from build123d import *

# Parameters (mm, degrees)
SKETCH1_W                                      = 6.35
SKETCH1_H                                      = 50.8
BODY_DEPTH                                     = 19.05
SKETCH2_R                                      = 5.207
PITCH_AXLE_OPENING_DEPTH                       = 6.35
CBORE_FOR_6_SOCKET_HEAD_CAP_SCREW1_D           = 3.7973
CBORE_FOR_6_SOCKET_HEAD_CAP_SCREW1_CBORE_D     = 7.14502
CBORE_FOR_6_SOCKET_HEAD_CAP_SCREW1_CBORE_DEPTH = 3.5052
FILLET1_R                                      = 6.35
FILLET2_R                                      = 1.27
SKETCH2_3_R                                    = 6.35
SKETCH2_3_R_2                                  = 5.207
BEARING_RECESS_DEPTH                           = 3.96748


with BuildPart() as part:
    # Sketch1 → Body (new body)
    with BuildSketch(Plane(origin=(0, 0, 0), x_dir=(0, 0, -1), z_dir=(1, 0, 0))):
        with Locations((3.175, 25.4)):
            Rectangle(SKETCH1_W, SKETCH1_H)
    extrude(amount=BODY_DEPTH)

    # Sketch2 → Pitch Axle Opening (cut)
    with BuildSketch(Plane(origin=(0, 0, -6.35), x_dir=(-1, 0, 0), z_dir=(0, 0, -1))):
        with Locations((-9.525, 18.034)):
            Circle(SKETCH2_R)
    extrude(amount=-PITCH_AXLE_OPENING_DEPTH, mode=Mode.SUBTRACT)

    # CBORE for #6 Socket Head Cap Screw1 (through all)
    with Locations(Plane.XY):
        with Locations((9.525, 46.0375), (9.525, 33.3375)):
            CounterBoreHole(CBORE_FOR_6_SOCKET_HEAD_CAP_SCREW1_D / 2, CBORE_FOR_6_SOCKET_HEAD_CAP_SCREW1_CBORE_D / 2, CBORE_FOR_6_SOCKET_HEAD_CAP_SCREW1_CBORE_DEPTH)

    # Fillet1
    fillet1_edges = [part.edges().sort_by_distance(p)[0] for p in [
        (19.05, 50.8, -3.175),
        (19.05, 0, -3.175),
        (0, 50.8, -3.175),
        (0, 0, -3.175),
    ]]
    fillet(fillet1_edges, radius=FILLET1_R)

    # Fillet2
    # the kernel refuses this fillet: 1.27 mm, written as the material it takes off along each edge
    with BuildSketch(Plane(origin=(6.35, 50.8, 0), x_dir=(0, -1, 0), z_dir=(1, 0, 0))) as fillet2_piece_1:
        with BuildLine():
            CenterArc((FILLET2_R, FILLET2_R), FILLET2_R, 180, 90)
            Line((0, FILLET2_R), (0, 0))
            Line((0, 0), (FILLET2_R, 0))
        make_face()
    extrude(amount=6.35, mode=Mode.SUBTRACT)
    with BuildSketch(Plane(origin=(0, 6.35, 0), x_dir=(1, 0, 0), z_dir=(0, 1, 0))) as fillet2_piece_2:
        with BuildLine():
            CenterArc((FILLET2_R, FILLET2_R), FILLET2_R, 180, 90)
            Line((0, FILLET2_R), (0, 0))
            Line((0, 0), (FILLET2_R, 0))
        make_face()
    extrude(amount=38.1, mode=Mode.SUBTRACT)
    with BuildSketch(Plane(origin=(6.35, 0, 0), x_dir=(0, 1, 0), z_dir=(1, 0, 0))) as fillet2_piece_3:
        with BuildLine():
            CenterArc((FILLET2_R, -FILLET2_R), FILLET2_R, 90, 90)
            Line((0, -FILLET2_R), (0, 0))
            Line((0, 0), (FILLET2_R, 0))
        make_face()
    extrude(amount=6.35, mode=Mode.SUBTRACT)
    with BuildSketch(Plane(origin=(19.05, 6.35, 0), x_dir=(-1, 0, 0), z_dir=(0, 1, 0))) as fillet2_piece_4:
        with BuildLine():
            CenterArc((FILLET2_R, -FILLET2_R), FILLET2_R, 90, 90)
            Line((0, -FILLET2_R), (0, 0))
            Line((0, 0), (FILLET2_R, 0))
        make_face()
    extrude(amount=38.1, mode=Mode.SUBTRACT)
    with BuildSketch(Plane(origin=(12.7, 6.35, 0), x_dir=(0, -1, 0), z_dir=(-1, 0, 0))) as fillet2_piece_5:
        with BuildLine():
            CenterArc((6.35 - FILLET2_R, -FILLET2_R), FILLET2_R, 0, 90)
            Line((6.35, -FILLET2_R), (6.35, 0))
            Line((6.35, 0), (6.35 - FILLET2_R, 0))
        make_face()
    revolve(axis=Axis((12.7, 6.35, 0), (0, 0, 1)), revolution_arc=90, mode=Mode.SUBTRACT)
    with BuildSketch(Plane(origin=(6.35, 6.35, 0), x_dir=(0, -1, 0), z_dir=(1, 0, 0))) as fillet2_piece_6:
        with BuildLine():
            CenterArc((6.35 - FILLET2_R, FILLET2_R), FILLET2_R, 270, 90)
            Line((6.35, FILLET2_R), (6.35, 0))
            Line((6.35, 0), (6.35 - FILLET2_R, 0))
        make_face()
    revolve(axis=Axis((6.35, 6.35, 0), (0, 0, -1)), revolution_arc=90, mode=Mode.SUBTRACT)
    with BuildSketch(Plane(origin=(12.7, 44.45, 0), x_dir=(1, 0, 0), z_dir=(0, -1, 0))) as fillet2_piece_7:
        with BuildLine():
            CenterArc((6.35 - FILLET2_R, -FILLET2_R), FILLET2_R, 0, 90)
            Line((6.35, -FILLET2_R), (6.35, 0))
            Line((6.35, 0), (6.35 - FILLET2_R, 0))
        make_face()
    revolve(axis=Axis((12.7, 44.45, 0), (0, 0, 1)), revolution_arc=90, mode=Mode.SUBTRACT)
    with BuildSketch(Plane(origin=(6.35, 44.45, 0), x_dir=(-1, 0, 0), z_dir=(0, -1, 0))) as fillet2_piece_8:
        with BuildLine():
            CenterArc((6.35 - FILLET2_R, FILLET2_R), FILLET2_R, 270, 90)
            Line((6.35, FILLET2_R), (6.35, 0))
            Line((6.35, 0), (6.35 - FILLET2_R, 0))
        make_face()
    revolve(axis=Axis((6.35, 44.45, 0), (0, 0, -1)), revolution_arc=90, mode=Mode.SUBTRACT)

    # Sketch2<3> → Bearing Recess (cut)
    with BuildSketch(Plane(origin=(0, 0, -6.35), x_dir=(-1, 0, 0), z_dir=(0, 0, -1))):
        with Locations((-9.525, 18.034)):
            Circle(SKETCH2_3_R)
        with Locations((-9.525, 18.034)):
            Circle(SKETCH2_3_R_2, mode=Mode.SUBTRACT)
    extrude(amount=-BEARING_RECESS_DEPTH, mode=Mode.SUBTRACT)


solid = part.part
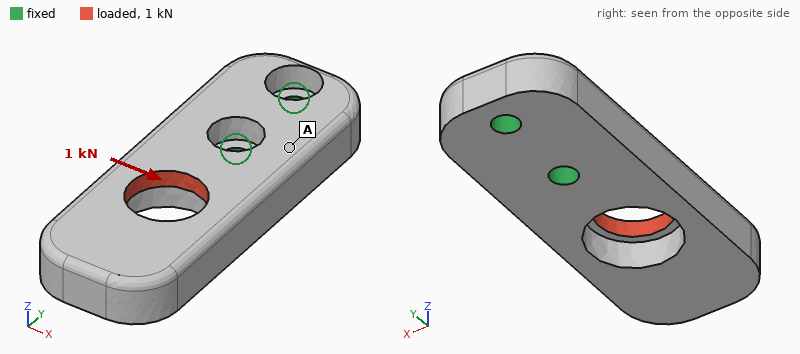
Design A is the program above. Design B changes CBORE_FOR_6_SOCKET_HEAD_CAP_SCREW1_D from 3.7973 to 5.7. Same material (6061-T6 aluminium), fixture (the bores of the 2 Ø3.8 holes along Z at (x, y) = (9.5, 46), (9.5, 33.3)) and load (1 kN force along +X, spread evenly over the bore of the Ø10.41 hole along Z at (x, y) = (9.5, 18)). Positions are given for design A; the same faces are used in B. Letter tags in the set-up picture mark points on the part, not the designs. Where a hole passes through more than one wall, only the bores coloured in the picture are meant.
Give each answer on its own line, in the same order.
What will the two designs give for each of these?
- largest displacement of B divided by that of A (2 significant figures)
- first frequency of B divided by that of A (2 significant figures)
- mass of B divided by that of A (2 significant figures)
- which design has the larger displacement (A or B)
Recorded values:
0.80
1.1
0.98
A
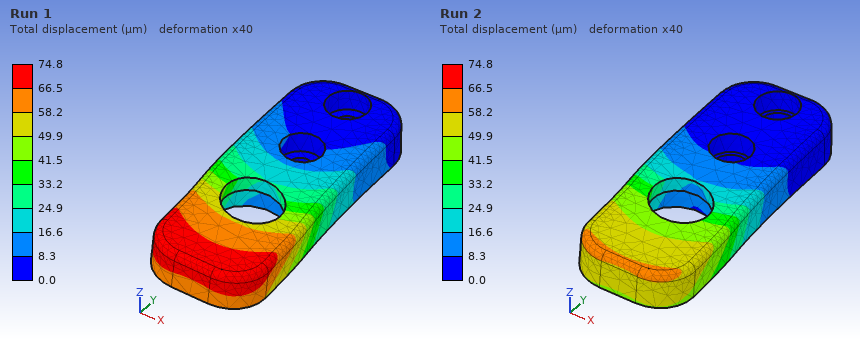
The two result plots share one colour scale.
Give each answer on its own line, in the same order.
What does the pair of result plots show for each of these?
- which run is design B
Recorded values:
Run 2
